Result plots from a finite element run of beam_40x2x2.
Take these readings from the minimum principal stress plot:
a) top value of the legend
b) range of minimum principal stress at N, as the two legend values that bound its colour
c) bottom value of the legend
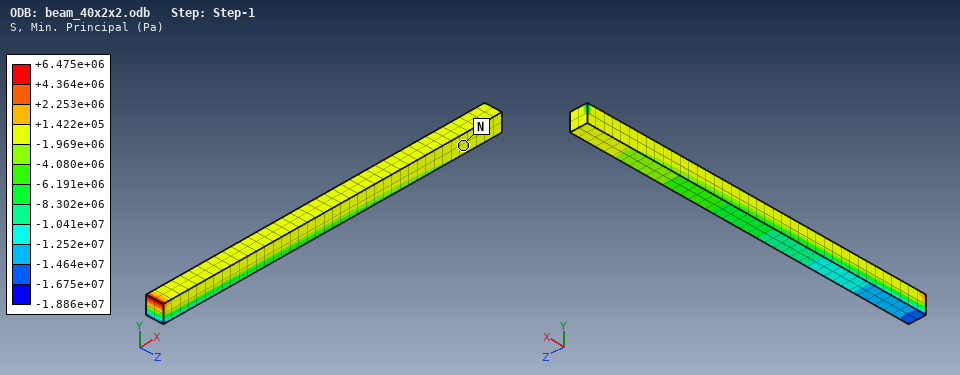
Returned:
+6.475e+06 Pa
-1.969e+06 to +1.422e+05 Pa
-1.886e+07 Pa
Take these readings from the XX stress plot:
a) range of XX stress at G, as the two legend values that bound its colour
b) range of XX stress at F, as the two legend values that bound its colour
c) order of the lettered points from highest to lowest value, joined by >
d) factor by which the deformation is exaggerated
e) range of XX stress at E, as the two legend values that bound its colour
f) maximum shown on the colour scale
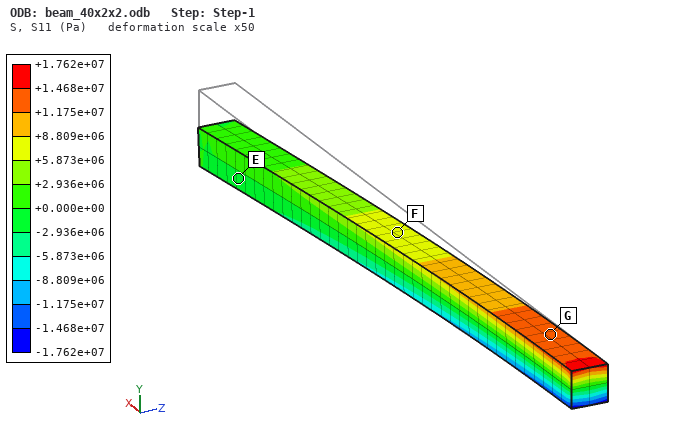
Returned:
+1.175e+07 to +1.468e+07 Pa
+5.873e+06 to +8.809e+06 Pa
G > F > E
50
-2.936e+06 to +0.000e+00 Pa
+1.762e+07 Pa
